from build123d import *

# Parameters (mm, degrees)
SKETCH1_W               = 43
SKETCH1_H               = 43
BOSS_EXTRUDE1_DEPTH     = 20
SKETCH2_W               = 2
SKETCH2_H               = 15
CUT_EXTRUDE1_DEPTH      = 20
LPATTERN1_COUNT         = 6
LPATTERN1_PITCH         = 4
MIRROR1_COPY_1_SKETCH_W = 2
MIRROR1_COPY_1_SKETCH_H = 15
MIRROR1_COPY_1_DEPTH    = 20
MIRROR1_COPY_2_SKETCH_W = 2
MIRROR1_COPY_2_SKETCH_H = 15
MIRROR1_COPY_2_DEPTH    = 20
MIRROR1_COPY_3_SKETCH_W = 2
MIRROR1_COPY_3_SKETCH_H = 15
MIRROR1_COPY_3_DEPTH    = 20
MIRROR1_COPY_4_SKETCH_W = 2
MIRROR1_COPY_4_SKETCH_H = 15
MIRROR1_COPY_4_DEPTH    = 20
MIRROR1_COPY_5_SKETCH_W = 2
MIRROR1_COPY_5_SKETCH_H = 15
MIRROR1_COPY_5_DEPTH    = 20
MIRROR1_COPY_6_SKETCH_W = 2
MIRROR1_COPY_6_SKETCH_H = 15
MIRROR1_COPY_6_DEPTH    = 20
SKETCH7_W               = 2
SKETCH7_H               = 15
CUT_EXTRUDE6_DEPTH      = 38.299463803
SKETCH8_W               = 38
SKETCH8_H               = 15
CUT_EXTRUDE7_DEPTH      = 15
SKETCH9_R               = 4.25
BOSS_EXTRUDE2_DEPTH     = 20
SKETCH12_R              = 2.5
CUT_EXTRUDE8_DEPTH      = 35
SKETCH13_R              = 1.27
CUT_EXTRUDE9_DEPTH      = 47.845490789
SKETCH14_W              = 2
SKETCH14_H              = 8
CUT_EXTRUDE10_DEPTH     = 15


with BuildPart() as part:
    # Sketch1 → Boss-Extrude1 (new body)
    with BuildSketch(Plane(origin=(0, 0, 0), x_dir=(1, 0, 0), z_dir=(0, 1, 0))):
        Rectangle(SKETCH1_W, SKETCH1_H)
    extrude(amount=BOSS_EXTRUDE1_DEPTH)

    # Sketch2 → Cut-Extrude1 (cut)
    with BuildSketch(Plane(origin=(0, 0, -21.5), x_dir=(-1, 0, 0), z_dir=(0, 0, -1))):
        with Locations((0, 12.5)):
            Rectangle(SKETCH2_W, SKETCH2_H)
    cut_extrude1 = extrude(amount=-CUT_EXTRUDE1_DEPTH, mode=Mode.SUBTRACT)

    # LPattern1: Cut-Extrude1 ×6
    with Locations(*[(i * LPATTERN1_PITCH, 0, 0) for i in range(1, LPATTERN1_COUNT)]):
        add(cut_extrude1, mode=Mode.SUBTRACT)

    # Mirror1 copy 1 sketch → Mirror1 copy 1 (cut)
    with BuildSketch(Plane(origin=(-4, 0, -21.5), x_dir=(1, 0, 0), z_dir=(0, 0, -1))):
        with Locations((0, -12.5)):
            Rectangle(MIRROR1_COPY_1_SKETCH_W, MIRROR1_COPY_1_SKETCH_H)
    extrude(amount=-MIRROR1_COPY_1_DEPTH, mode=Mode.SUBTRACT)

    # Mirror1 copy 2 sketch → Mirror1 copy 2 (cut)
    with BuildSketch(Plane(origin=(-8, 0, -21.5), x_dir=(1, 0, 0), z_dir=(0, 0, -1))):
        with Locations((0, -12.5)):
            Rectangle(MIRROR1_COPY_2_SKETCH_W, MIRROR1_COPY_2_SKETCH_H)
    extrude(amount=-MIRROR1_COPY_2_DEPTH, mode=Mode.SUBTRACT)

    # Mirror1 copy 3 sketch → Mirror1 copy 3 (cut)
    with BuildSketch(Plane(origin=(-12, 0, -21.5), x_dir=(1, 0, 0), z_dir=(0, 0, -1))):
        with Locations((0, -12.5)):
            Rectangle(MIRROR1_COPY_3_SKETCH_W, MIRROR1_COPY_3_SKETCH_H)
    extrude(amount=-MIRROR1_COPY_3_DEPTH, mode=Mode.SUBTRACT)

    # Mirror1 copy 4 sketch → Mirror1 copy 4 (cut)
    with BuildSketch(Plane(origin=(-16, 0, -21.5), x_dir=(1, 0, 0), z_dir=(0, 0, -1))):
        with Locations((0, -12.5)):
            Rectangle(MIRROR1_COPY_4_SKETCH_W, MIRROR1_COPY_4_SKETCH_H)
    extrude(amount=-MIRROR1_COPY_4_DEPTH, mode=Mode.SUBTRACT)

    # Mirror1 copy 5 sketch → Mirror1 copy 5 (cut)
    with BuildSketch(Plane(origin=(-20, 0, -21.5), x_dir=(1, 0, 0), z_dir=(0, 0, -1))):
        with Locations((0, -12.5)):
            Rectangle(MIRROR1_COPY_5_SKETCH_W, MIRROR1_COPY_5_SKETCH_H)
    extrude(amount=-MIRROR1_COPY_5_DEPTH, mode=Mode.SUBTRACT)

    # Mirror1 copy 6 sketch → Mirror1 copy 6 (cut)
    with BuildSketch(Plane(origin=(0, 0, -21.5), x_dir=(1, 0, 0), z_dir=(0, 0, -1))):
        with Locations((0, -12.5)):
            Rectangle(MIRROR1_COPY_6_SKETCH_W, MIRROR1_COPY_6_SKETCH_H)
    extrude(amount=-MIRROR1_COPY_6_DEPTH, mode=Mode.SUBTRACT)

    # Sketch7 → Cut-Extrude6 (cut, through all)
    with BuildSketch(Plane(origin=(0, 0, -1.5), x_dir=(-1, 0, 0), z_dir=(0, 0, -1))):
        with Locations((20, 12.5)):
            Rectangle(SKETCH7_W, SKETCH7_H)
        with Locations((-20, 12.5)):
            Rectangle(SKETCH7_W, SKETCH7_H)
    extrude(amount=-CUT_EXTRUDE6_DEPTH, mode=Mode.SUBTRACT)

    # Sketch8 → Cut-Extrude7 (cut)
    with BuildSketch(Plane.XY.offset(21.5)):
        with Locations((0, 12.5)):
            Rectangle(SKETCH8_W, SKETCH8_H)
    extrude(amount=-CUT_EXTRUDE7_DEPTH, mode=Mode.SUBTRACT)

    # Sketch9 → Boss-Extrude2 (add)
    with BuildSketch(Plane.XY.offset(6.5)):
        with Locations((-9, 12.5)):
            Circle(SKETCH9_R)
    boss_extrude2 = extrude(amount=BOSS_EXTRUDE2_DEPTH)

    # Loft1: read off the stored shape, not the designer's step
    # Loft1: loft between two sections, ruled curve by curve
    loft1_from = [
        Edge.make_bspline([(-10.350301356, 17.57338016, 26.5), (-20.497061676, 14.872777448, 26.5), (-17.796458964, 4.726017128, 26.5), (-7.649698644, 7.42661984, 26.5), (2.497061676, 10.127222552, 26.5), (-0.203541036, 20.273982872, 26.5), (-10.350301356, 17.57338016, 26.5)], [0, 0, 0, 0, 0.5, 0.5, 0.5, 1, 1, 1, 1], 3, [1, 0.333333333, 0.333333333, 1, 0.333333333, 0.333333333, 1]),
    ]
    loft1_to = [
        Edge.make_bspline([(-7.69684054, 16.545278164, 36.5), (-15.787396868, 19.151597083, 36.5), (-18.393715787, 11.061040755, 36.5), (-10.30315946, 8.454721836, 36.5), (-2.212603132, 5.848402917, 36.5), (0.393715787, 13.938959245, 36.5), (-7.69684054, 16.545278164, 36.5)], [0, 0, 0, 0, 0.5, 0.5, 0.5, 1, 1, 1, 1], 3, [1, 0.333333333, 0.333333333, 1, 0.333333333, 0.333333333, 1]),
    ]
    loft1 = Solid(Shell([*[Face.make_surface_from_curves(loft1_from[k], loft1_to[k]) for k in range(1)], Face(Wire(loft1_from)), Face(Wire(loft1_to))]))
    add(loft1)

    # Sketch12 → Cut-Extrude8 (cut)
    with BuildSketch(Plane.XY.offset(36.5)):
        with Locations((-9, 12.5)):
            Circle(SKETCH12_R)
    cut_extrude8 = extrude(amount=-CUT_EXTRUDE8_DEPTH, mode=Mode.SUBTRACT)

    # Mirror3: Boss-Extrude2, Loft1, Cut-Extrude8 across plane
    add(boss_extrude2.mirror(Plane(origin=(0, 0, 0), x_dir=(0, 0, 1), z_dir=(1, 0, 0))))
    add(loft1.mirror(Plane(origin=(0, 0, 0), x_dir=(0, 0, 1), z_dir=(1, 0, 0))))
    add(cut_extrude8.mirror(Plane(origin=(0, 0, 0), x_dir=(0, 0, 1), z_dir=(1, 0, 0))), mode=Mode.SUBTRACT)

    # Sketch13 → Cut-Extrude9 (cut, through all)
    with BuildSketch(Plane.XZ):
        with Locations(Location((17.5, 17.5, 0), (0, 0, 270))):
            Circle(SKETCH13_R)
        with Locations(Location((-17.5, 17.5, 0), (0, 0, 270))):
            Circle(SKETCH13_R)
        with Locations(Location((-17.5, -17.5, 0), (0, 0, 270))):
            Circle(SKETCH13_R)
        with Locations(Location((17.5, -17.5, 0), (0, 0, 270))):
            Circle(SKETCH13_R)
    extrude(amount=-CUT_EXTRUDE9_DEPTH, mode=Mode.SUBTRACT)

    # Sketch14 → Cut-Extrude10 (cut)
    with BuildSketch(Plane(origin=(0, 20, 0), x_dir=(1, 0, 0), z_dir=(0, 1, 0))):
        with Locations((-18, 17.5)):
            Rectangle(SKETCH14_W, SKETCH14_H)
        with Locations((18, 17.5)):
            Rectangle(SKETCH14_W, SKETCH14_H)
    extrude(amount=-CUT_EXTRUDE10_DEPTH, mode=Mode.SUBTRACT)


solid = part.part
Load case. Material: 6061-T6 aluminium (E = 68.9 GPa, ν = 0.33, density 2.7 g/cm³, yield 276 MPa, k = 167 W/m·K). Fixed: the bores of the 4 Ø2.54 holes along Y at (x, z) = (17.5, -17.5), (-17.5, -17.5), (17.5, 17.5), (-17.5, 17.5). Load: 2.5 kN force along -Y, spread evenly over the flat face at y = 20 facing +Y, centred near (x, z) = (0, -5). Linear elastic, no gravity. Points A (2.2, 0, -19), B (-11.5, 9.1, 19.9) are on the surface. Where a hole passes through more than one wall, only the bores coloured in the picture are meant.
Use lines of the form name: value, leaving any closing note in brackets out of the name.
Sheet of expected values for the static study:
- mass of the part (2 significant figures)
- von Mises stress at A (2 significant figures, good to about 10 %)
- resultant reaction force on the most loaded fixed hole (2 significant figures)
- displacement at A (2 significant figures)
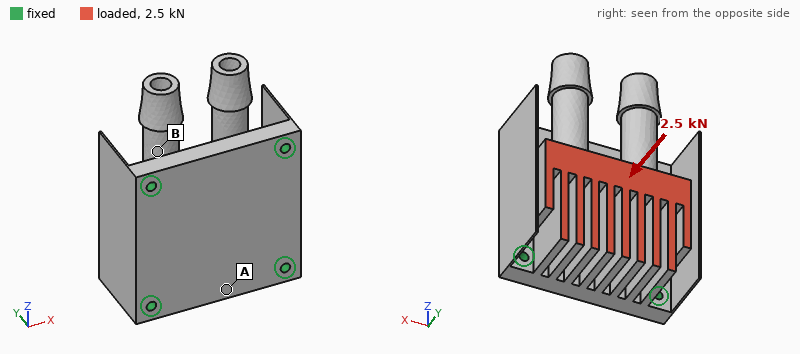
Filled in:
mass of the part: 60 g
von Mises stress at A: 15 MPa
resultant reaction force on the most loaded fixed hole: 810 N
displacement at A: 12 µm
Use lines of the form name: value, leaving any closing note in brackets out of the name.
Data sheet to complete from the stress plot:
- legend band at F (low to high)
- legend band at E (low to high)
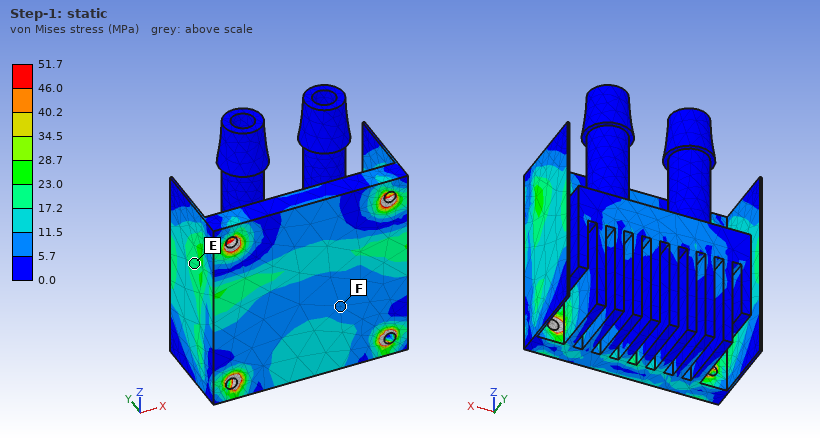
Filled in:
legend band at F: 5.7 to 11.5 MPa
legend band at E: 17.2 to 23.0 MPa
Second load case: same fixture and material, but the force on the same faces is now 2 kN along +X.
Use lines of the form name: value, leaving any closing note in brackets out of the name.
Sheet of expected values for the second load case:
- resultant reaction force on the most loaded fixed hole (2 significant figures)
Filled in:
resultant reaction force on the most loaded fixed hole: 830 N
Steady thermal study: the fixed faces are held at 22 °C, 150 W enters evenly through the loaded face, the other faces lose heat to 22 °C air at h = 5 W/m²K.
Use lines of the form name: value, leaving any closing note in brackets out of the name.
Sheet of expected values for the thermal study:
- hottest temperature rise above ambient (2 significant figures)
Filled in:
hottest temperature rise above ambient: 54 K
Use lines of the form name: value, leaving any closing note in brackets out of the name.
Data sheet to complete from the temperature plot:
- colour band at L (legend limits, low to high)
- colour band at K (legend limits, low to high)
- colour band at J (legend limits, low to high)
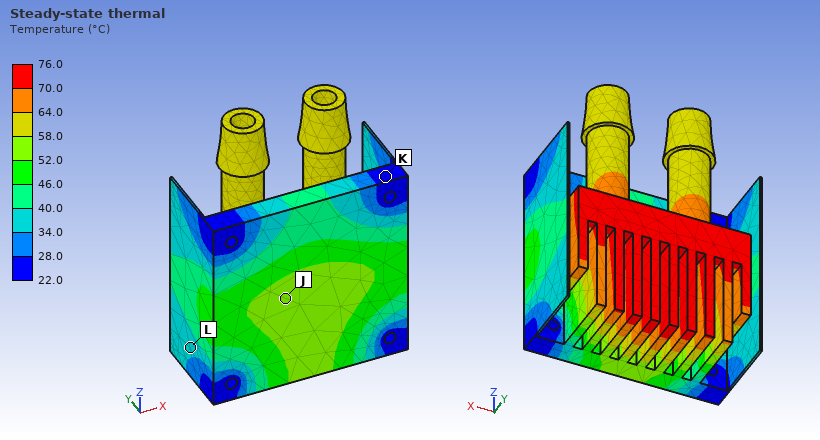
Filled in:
colour band at L: 34.0 to 40.0 °C
colour band at K: 22.0 to 28.0 °C
colour band at J: 52.0 to 58.0 °C
